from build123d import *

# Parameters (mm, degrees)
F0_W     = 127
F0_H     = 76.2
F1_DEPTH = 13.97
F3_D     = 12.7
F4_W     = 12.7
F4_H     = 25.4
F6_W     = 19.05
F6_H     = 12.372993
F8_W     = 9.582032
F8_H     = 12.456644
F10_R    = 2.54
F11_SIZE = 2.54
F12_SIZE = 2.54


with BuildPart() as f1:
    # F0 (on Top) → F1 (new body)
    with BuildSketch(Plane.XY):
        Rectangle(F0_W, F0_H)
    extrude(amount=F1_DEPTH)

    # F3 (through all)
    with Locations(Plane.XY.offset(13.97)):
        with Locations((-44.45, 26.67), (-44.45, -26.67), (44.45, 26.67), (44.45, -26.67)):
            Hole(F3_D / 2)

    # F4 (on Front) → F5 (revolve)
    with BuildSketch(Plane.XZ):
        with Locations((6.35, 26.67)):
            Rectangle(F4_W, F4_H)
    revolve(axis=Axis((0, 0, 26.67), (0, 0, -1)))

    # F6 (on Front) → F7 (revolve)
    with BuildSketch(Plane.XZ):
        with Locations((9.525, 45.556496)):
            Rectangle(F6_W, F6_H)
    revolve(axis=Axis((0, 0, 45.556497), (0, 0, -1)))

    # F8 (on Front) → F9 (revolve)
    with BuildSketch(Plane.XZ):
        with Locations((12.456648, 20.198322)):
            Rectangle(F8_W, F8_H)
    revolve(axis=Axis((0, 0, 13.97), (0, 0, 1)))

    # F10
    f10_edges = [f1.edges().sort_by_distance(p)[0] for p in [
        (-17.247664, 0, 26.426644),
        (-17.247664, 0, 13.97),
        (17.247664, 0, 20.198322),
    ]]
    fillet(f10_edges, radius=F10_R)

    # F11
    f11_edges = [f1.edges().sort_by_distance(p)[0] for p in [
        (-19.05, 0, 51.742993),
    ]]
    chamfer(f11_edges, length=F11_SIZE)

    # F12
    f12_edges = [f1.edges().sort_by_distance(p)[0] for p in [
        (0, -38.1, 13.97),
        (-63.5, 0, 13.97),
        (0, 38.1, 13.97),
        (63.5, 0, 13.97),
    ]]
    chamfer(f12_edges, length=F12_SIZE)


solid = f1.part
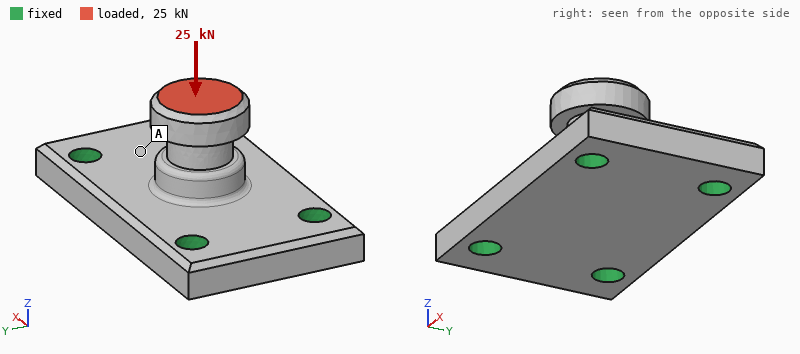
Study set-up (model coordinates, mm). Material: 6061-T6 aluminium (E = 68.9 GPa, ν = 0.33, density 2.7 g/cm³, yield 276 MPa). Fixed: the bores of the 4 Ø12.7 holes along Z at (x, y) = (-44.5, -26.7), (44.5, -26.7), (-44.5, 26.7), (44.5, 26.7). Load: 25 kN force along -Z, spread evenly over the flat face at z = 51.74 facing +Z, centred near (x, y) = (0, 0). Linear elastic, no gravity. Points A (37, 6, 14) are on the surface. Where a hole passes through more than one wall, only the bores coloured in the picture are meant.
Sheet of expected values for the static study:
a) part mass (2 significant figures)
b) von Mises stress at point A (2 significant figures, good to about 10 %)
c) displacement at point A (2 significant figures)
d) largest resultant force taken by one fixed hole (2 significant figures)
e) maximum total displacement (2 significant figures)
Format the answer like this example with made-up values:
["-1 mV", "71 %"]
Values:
["430 g", "26 MPa", "19 µm", "6.4 kN", "88 µm"]
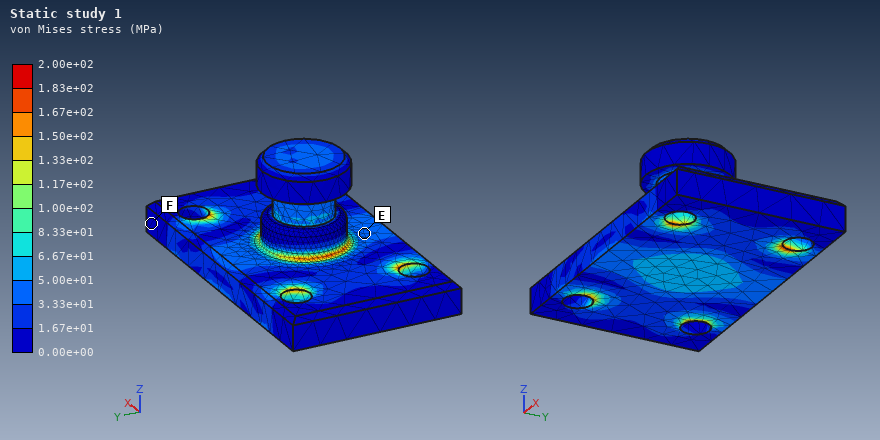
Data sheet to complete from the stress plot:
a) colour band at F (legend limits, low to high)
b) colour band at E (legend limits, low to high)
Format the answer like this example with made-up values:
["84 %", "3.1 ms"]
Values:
["0.00e+00 to 1.67e+01 MPa", "3.33e+01 to 5.00e+01 MPa"]
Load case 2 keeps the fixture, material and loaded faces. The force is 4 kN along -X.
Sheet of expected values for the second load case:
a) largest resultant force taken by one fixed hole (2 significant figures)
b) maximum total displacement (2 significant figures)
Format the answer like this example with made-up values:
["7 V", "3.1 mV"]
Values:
["1.7 kN", "74 µm"]
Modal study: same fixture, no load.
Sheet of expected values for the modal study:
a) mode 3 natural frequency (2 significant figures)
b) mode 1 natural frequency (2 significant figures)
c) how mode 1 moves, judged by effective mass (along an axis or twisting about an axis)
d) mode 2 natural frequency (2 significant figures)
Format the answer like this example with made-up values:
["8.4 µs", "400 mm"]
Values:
["6900 Hz", "5700 Hz", "along Y", "6700 Hz"]
